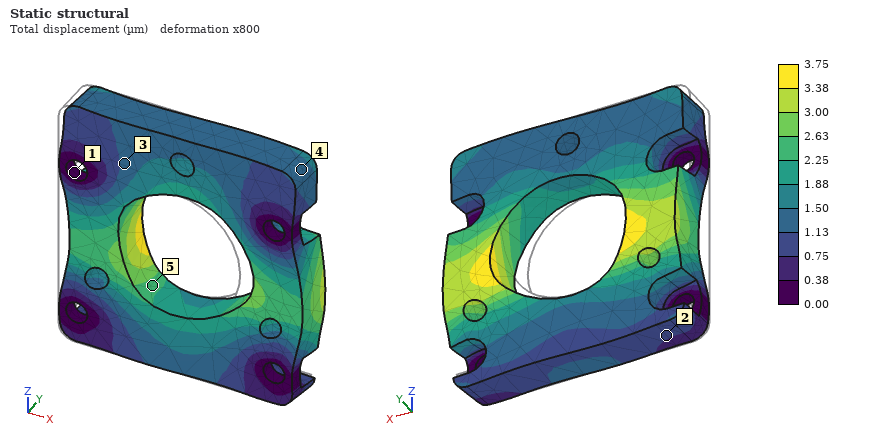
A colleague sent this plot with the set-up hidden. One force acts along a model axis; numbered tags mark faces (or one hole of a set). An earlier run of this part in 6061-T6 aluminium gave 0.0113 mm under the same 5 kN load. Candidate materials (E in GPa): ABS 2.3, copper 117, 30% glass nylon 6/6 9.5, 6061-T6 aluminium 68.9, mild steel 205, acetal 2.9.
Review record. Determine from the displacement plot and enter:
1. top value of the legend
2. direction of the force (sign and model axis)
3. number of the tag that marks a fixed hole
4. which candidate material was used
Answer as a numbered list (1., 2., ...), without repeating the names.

1. 3.75 µm
2. +X
3. 1
4. mild steel
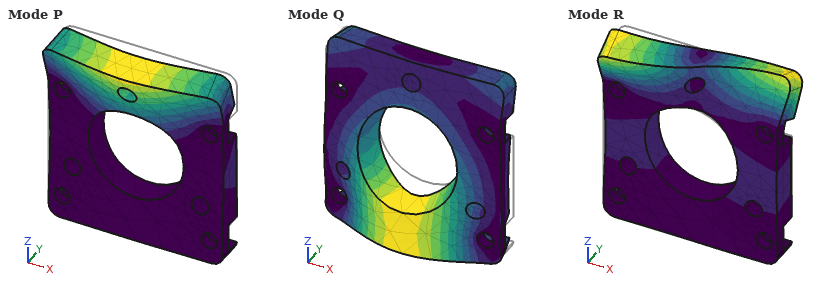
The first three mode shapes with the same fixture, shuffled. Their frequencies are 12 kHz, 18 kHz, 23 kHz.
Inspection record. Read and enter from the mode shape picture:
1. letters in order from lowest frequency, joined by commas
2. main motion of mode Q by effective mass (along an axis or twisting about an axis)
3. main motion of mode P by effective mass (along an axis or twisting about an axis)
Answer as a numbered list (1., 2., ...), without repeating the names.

1. P, Q, R
2. along Y
3. along Y
